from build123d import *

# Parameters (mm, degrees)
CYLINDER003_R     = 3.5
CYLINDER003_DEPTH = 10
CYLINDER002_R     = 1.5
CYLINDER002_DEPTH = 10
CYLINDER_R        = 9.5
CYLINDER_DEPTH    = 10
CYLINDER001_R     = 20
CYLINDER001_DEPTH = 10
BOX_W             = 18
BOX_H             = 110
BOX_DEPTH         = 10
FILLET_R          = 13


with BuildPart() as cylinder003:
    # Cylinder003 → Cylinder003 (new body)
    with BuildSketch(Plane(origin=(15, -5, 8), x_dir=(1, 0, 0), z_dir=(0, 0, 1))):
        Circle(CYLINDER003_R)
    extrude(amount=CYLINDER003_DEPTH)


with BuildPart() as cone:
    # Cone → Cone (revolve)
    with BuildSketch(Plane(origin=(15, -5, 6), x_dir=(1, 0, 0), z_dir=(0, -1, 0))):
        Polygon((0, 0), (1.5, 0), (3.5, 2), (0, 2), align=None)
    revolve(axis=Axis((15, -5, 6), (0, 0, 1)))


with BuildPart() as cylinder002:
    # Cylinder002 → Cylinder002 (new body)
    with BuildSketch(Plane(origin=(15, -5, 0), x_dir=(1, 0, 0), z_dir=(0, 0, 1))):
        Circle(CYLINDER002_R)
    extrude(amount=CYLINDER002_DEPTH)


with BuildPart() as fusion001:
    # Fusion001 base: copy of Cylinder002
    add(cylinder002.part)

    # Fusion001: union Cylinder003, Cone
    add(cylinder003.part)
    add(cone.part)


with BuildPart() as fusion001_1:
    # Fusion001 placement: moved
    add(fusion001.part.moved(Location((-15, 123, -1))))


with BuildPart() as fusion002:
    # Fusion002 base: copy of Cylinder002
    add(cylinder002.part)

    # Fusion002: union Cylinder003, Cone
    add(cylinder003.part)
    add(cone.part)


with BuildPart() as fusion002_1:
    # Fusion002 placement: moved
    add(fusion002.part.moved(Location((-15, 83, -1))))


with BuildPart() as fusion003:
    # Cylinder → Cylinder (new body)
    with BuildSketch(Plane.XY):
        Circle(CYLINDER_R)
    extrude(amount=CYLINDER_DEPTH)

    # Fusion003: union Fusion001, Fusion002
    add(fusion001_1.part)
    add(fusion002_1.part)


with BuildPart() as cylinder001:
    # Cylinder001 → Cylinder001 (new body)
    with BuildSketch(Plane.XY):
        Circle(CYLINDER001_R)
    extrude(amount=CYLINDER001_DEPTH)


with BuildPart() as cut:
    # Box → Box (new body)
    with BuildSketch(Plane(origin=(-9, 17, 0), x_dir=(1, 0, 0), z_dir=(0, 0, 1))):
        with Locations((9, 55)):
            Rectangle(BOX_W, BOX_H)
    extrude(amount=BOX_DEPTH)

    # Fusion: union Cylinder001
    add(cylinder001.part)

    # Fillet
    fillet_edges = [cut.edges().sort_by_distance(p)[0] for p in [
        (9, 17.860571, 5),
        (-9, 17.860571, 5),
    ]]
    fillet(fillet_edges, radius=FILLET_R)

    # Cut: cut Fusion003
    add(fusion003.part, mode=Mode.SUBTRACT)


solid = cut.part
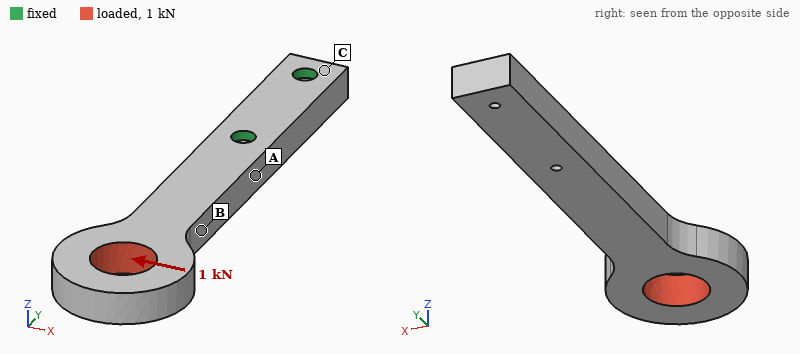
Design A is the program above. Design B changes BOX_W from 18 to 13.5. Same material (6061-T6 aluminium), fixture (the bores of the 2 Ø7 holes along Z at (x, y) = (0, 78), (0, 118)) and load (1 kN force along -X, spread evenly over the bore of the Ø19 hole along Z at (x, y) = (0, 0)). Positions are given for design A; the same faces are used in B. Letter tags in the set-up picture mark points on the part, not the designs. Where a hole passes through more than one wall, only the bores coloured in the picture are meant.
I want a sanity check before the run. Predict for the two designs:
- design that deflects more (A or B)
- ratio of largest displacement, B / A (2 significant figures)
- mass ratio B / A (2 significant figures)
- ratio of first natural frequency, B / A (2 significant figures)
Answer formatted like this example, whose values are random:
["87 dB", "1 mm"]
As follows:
["B", "2.1", "0.83", "0.89"]
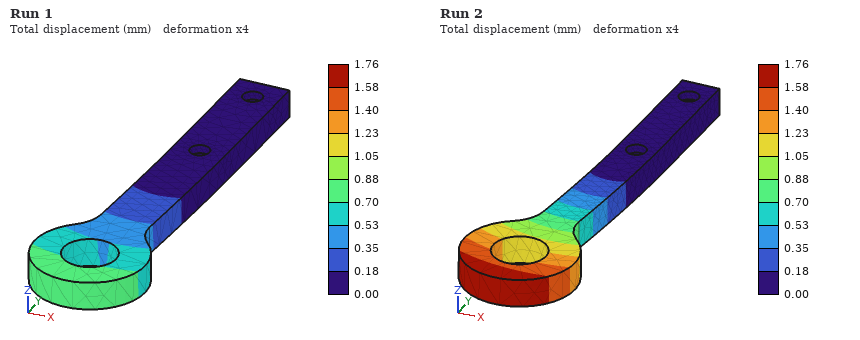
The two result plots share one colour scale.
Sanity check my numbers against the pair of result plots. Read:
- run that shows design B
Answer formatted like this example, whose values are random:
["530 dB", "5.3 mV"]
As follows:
["Run 2"]
